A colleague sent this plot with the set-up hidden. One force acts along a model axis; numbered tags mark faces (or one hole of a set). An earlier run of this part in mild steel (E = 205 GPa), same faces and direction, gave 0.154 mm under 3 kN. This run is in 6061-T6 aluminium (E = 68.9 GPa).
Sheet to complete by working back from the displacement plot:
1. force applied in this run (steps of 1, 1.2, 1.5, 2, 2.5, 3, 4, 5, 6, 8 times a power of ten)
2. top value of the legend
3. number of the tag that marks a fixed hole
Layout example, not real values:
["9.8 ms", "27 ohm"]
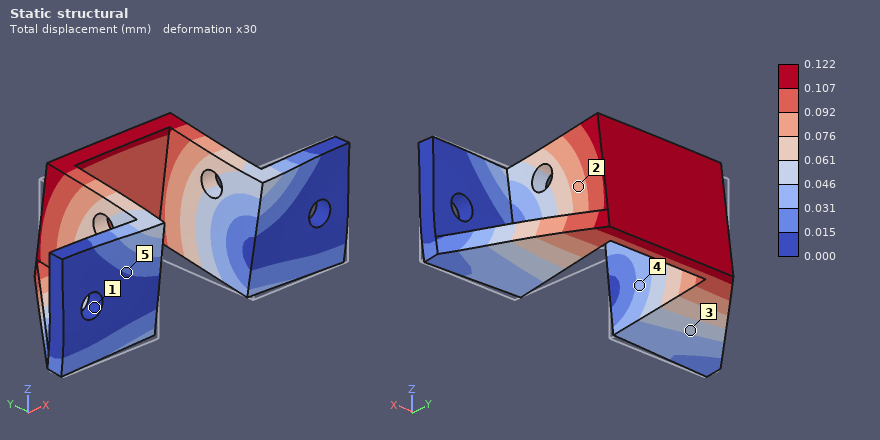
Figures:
["800 N", "0.122 mm", "1"]
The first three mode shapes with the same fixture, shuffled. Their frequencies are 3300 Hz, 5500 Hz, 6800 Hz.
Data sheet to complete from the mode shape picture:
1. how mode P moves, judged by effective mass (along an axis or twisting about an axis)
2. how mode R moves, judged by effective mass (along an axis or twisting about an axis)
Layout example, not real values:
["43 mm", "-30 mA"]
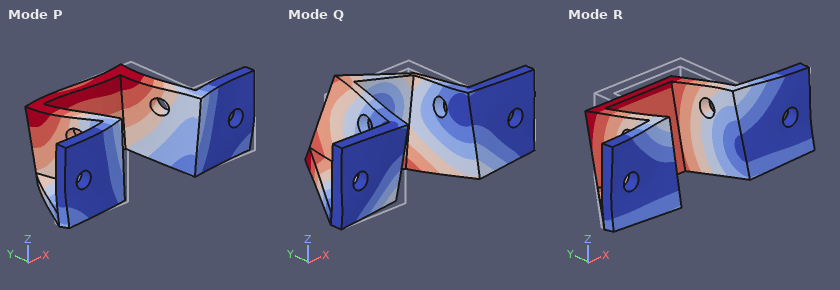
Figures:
["along X", "along Z"]
